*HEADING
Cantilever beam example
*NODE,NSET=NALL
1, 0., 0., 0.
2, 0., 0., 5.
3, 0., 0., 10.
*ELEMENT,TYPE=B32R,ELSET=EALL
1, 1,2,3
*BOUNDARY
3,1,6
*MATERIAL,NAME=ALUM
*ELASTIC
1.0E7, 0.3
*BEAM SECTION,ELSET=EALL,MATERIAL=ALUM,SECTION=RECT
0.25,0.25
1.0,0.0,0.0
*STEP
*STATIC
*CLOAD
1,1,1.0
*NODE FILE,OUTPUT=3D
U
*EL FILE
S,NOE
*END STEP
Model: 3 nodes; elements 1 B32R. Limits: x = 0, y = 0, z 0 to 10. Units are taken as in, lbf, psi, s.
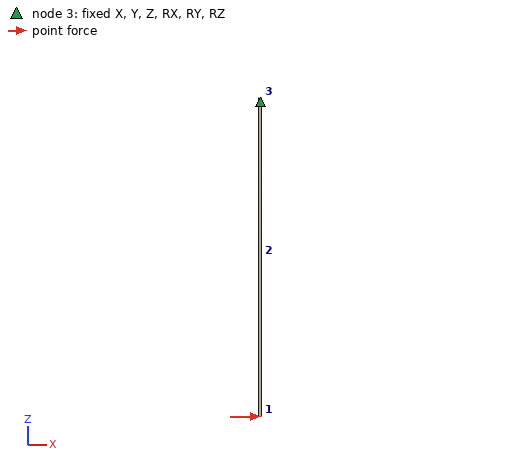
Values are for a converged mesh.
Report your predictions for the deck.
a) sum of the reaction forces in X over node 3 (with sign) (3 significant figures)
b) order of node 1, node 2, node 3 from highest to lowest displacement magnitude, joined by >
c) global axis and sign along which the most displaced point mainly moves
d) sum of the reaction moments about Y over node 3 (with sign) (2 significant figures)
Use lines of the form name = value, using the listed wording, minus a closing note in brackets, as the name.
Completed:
sum of the reaction forces in X over node 3 (with sign) = -1.00 lbf
order of node 1, node 2, node 3 from highest to lowest displacement magnitude, joined by > = node 1 > node 2 > node 3
global axis and sign along which the most displaced point mainly moves = +X
sum of the reaction moments about Y over node 3 (with sign) = 10 lbf·in
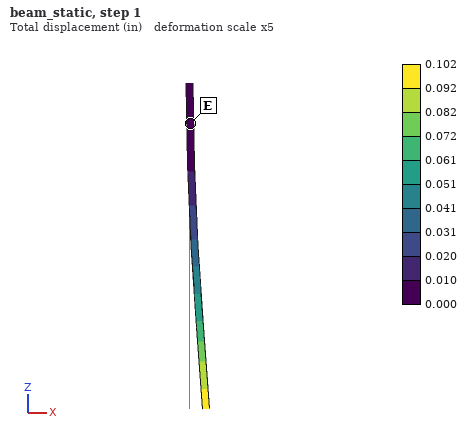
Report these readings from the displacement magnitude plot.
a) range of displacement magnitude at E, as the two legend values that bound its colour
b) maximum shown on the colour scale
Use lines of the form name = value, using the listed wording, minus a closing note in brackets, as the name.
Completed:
range of displacement magnitude at E, as the two legend values that bound its colour = 0.000 to 0.010 in
maximum shown on the colour scale = 0.102 in
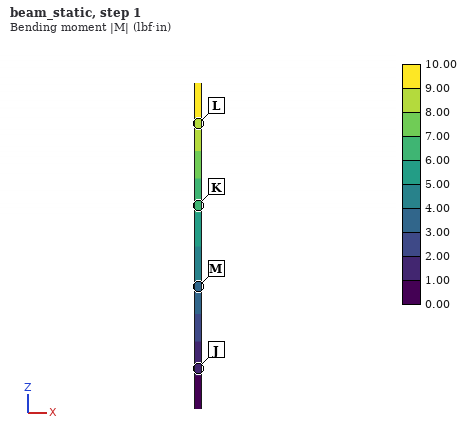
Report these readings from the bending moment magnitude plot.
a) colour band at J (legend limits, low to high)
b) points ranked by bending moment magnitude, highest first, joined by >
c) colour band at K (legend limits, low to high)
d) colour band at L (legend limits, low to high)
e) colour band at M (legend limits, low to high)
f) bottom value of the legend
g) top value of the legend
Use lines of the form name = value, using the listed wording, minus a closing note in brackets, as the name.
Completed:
colour band at J = 1.00 to 2.00 lbf·in
points ranked by bending moment magnitude, highest first, joined by > = L > K > M > J
colour band at K = 6.00 to 7.00 lbf·in
colour band at L = 8.00 to 9.00 lbf·in
colour band at M = 3.00 to 4.00 lbf·in
bottom value of the legend = 0.00 lbf·in
top value of the legend = 10.00 lbf·in
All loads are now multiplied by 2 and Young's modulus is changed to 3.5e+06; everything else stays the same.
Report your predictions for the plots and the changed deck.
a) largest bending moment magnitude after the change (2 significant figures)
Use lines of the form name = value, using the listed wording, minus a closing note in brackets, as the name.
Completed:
largest bending moment magnitude after the change = 20 lbf·in
